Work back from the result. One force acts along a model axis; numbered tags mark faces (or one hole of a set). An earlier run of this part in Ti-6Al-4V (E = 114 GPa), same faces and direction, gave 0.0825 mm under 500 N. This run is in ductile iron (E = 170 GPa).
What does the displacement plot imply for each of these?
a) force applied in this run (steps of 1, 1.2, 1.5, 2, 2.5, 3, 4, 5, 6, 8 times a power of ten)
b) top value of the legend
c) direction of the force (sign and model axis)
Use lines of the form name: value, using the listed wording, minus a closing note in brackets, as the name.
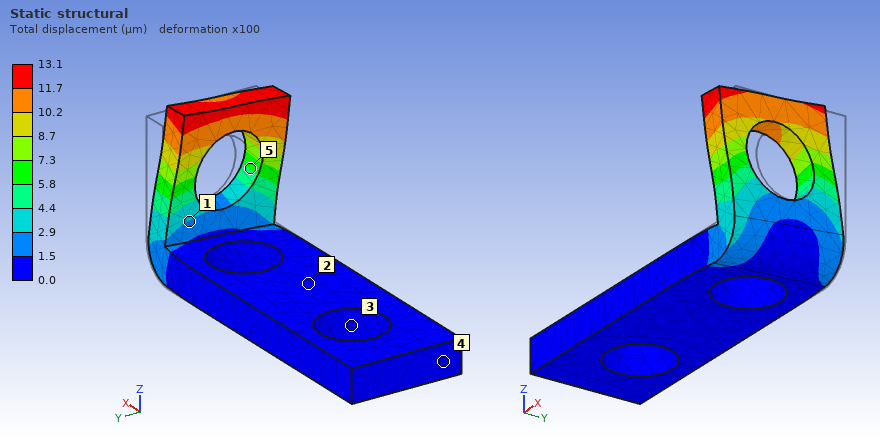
force applied in this run: 120 N
top value of the legend: 13.1 µm
direction of the force: -Y
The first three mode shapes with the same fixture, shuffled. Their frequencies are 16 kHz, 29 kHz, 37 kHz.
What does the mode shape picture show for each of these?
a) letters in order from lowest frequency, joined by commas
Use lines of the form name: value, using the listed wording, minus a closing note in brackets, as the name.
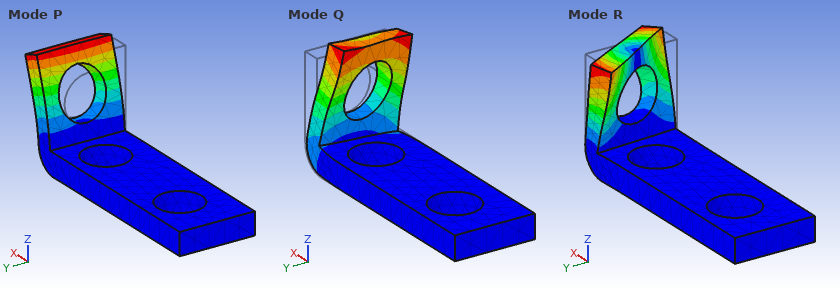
letters in order from lowest frequency, joined by commas: P, Q, R
